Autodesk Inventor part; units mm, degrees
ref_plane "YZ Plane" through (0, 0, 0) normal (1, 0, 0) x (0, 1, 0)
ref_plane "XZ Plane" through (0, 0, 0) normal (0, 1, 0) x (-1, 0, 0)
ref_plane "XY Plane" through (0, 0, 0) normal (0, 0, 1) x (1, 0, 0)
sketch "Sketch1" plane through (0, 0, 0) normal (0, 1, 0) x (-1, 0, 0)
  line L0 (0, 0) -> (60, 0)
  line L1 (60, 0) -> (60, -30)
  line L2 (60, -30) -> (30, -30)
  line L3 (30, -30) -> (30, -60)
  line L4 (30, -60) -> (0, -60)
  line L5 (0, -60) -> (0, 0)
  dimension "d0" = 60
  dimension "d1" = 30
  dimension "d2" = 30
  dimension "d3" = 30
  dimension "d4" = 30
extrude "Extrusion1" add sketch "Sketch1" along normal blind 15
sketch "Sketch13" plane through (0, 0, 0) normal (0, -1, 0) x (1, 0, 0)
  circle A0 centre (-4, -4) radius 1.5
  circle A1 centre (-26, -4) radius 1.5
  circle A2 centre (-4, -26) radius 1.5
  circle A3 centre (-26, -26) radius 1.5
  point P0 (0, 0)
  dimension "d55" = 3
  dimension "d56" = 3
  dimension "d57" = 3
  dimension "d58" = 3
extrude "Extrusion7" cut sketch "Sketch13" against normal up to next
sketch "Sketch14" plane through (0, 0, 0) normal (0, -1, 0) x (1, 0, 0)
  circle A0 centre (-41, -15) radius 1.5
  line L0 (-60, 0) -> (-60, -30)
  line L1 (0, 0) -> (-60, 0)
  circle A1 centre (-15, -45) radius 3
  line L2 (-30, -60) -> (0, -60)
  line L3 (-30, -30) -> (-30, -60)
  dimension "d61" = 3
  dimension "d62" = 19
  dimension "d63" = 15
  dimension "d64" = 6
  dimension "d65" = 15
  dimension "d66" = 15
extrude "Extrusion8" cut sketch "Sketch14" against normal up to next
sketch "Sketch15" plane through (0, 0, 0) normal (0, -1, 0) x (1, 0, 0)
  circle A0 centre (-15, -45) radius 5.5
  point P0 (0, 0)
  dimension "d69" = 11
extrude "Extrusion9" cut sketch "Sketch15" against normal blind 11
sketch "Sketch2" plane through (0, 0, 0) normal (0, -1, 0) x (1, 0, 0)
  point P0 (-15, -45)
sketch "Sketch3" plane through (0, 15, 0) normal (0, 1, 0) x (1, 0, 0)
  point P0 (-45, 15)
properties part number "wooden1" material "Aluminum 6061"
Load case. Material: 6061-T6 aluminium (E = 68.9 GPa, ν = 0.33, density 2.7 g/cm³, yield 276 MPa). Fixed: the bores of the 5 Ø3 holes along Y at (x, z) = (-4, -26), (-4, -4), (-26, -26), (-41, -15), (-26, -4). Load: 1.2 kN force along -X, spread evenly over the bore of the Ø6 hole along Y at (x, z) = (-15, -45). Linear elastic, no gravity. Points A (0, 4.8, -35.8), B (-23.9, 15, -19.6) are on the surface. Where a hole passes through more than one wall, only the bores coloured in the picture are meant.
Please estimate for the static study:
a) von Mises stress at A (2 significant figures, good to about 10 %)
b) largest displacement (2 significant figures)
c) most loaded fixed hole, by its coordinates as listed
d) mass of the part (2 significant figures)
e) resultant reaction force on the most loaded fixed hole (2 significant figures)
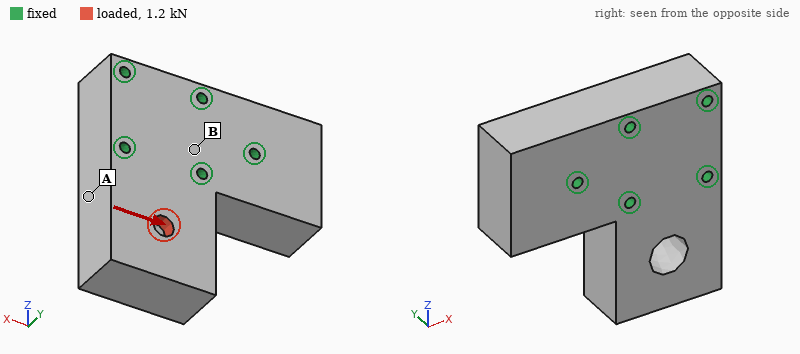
7.4 MPa
7.6 µm
(-4, -26)
100 g
1.1 kN
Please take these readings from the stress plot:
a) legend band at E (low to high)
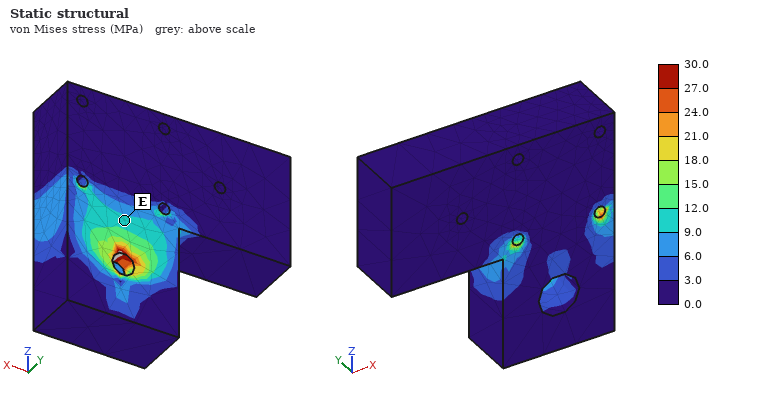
9.0 to 12.0 MPa
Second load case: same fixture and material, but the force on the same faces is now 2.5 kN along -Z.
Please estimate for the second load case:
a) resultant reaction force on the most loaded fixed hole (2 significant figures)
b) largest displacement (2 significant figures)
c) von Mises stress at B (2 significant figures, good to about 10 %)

1.1 kN
14 µm
4.1 MPa
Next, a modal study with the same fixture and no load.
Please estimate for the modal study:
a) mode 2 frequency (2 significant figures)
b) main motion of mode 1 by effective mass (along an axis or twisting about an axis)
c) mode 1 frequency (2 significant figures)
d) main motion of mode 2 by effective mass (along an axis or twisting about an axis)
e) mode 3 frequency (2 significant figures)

14 kHz
along Y
8600 Hz
along X
17 kHz
